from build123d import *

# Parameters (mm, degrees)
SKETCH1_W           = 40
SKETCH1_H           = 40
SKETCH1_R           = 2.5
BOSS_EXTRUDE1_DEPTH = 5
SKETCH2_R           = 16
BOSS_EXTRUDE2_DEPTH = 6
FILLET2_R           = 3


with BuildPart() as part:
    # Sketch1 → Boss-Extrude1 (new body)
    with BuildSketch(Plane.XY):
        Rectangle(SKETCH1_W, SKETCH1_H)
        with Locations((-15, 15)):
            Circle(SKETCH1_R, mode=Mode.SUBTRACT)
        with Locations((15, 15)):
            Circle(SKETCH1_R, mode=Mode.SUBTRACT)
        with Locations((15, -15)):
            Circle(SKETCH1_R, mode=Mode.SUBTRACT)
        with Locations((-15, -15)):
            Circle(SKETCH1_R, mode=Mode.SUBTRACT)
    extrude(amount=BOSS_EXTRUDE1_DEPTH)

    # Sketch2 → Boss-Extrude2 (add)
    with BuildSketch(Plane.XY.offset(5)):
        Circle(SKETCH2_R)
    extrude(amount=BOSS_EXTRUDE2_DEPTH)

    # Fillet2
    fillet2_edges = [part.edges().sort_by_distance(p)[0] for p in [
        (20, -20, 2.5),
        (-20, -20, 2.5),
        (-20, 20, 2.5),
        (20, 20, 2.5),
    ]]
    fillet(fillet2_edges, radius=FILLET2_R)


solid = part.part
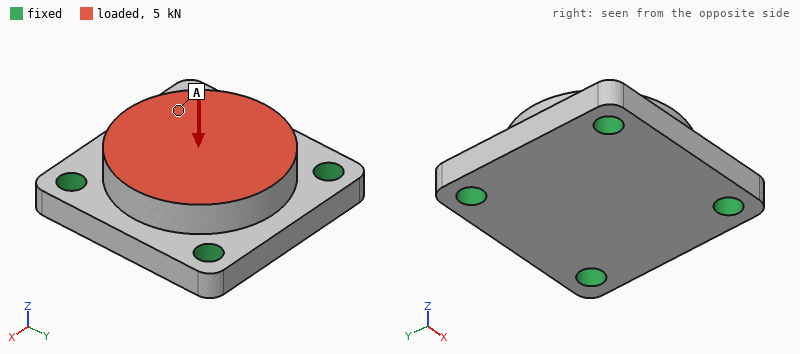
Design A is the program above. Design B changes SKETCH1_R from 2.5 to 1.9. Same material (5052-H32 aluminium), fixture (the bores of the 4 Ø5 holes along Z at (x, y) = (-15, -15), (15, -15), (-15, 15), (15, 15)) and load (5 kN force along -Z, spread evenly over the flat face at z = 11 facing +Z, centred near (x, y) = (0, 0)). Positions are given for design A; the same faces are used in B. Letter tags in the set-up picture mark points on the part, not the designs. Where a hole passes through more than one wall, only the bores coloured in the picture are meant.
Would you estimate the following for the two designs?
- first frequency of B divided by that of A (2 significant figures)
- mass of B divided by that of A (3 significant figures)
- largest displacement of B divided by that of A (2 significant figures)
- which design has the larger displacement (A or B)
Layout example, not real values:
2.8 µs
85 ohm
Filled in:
0.90
1.01
1.2
B
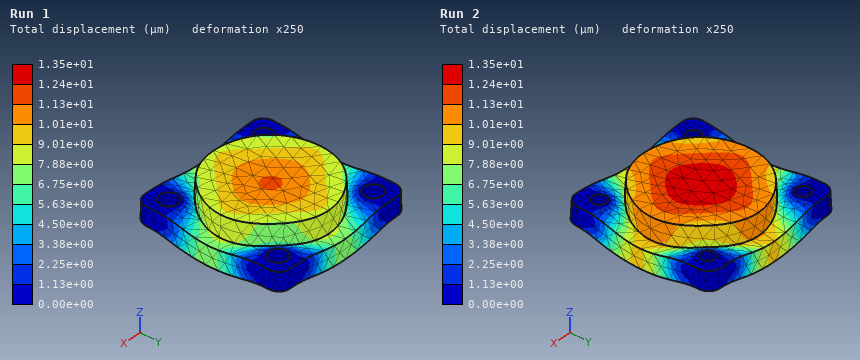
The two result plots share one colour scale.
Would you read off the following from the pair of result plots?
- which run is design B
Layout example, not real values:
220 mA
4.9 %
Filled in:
Run 2
